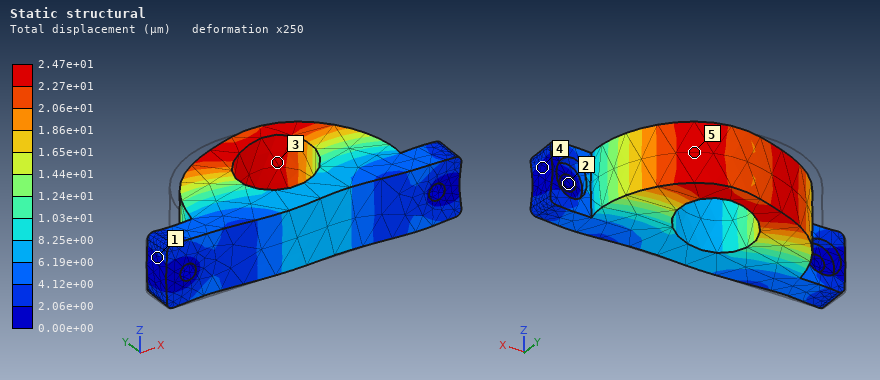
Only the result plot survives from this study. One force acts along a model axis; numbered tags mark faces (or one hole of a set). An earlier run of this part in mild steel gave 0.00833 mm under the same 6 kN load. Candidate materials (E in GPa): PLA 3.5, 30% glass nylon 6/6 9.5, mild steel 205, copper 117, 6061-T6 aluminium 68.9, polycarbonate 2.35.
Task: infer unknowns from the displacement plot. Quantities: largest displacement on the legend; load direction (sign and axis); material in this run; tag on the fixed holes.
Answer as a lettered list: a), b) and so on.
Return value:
a) 2.47e+01 µm
b) +X
c) 6061-T6 aluminium
d) 2
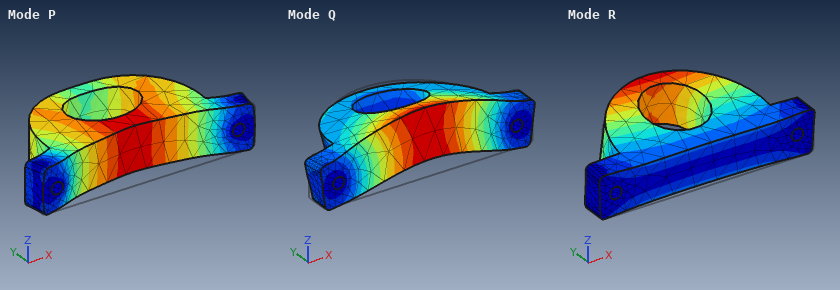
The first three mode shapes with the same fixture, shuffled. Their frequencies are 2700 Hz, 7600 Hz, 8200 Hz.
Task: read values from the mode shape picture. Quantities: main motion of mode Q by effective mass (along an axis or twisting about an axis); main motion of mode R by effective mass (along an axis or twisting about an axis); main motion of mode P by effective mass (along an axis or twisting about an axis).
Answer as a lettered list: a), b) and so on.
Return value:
a) along Z
b) along Z
c) along Y
